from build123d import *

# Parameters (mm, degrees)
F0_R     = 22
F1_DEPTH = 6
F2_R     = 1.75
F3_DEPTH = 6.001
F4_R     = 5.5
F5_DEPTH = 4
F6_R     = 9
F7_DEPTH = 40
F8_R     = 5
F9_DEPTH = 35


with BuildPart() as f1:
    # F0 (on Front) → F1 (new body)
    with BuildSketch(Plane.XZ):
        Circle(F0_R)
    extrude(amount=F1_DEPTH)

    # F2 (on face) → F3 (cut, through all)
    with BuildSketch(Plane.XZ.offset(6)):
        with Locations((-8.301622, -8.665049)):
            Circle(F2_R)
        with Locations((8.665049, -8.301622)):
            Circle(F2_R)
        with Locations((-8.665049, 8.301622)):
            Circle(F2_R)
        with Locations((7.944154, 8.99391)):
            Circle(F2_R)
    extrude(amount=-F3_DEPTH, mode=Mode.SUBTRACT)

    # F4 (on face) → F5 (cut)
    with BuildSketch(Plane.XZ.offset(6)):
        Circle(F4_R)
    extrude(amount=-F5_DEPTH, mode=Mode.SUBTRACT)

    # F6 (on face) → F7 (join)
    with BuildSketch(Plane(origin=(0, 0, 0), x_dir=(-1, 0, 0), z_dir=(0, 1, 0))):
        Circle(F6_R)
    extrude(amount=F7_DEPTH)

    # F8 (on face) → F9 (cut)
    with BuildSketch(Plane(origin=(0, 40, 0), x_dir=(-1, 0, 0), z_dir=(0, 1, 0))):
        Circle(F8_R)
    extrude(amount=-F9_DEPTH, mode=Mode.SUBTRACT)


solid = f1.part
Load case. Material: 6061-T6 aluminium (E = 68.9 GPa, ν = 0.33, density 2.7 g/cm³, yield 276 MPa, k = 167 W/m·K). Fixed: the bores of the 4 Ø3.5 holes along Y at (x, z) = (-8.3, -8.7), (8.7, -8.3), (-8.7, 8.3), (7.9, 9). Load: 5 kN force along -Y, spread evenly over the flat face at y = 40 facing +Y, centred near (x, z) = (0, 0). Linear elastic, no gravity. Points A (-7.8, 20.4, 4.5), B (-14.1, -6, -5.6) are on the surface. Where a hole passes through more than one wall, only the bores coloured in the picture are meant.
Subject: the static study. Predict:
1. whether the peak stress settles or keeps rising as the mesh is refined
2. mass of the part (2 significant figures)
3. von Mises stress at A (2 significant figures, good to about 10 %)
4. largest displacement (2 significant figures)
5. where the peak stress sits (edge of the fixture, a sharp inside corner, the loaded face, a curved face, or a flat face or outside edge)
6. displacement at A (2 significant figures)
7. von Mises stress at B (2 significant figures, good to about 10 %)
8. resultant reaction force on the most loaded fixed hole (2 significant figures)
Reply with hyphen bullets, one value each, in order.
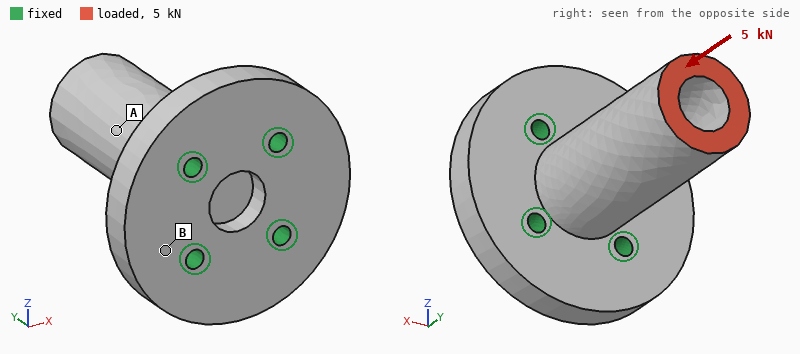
- keeps rising
- 43 g
- 29 MPa
- 21 µm
- edge of the fixture
- 12 µm
- 9.1 MPa
- 1.4 kN
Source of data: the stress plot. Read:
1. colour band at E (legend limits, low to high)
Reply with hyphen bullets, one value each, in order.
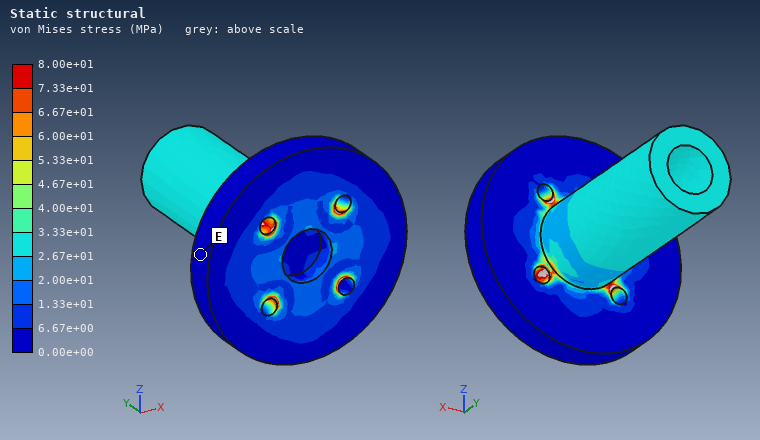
- 0.00e+00 to 6.67e+00 MPa
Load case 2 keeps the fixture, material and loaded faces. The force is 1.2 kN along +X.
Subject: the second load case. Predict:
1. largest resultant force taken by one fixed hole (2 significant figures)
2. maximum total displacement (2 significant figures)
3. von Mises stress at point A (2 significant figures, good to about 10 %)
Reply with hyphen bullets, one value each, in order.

- 1.7 kN
- 0.14 mm
- 40 MPa
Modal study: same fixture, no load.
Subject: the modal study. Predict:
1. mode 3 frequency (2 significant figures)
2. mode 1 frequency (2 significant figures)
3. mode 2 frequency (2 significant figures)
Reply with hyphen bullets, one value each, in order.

- 18 kHz
- 6400 Hz
- 6400 Hz
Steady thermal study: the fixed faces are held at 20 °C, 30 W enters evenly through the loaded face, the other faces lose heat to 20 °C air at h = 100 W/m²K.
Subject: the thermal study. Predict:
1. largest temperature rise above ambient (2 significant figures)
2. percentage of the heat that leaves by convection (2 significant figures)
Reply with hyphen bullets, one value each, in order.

- 37 K
- 23 %
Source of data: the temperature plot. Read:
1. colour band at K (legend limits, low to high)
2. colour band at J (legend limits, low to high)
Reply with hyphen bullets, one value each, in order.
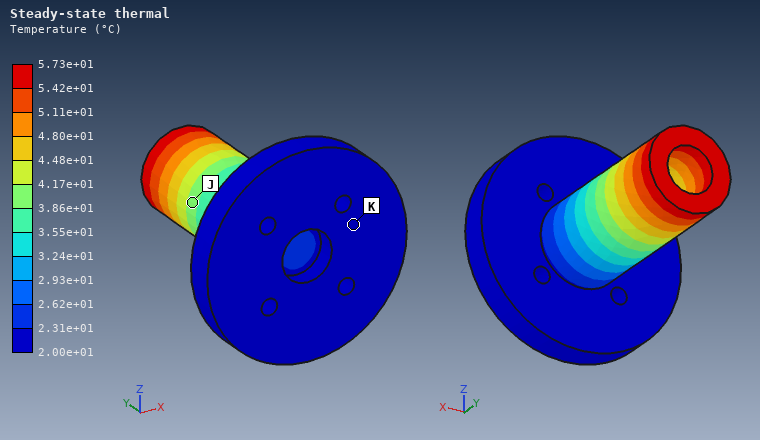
- 2.00e+01 to 2.31e+01 °C
- 3.86e+01 to 4.17e+01 °C
